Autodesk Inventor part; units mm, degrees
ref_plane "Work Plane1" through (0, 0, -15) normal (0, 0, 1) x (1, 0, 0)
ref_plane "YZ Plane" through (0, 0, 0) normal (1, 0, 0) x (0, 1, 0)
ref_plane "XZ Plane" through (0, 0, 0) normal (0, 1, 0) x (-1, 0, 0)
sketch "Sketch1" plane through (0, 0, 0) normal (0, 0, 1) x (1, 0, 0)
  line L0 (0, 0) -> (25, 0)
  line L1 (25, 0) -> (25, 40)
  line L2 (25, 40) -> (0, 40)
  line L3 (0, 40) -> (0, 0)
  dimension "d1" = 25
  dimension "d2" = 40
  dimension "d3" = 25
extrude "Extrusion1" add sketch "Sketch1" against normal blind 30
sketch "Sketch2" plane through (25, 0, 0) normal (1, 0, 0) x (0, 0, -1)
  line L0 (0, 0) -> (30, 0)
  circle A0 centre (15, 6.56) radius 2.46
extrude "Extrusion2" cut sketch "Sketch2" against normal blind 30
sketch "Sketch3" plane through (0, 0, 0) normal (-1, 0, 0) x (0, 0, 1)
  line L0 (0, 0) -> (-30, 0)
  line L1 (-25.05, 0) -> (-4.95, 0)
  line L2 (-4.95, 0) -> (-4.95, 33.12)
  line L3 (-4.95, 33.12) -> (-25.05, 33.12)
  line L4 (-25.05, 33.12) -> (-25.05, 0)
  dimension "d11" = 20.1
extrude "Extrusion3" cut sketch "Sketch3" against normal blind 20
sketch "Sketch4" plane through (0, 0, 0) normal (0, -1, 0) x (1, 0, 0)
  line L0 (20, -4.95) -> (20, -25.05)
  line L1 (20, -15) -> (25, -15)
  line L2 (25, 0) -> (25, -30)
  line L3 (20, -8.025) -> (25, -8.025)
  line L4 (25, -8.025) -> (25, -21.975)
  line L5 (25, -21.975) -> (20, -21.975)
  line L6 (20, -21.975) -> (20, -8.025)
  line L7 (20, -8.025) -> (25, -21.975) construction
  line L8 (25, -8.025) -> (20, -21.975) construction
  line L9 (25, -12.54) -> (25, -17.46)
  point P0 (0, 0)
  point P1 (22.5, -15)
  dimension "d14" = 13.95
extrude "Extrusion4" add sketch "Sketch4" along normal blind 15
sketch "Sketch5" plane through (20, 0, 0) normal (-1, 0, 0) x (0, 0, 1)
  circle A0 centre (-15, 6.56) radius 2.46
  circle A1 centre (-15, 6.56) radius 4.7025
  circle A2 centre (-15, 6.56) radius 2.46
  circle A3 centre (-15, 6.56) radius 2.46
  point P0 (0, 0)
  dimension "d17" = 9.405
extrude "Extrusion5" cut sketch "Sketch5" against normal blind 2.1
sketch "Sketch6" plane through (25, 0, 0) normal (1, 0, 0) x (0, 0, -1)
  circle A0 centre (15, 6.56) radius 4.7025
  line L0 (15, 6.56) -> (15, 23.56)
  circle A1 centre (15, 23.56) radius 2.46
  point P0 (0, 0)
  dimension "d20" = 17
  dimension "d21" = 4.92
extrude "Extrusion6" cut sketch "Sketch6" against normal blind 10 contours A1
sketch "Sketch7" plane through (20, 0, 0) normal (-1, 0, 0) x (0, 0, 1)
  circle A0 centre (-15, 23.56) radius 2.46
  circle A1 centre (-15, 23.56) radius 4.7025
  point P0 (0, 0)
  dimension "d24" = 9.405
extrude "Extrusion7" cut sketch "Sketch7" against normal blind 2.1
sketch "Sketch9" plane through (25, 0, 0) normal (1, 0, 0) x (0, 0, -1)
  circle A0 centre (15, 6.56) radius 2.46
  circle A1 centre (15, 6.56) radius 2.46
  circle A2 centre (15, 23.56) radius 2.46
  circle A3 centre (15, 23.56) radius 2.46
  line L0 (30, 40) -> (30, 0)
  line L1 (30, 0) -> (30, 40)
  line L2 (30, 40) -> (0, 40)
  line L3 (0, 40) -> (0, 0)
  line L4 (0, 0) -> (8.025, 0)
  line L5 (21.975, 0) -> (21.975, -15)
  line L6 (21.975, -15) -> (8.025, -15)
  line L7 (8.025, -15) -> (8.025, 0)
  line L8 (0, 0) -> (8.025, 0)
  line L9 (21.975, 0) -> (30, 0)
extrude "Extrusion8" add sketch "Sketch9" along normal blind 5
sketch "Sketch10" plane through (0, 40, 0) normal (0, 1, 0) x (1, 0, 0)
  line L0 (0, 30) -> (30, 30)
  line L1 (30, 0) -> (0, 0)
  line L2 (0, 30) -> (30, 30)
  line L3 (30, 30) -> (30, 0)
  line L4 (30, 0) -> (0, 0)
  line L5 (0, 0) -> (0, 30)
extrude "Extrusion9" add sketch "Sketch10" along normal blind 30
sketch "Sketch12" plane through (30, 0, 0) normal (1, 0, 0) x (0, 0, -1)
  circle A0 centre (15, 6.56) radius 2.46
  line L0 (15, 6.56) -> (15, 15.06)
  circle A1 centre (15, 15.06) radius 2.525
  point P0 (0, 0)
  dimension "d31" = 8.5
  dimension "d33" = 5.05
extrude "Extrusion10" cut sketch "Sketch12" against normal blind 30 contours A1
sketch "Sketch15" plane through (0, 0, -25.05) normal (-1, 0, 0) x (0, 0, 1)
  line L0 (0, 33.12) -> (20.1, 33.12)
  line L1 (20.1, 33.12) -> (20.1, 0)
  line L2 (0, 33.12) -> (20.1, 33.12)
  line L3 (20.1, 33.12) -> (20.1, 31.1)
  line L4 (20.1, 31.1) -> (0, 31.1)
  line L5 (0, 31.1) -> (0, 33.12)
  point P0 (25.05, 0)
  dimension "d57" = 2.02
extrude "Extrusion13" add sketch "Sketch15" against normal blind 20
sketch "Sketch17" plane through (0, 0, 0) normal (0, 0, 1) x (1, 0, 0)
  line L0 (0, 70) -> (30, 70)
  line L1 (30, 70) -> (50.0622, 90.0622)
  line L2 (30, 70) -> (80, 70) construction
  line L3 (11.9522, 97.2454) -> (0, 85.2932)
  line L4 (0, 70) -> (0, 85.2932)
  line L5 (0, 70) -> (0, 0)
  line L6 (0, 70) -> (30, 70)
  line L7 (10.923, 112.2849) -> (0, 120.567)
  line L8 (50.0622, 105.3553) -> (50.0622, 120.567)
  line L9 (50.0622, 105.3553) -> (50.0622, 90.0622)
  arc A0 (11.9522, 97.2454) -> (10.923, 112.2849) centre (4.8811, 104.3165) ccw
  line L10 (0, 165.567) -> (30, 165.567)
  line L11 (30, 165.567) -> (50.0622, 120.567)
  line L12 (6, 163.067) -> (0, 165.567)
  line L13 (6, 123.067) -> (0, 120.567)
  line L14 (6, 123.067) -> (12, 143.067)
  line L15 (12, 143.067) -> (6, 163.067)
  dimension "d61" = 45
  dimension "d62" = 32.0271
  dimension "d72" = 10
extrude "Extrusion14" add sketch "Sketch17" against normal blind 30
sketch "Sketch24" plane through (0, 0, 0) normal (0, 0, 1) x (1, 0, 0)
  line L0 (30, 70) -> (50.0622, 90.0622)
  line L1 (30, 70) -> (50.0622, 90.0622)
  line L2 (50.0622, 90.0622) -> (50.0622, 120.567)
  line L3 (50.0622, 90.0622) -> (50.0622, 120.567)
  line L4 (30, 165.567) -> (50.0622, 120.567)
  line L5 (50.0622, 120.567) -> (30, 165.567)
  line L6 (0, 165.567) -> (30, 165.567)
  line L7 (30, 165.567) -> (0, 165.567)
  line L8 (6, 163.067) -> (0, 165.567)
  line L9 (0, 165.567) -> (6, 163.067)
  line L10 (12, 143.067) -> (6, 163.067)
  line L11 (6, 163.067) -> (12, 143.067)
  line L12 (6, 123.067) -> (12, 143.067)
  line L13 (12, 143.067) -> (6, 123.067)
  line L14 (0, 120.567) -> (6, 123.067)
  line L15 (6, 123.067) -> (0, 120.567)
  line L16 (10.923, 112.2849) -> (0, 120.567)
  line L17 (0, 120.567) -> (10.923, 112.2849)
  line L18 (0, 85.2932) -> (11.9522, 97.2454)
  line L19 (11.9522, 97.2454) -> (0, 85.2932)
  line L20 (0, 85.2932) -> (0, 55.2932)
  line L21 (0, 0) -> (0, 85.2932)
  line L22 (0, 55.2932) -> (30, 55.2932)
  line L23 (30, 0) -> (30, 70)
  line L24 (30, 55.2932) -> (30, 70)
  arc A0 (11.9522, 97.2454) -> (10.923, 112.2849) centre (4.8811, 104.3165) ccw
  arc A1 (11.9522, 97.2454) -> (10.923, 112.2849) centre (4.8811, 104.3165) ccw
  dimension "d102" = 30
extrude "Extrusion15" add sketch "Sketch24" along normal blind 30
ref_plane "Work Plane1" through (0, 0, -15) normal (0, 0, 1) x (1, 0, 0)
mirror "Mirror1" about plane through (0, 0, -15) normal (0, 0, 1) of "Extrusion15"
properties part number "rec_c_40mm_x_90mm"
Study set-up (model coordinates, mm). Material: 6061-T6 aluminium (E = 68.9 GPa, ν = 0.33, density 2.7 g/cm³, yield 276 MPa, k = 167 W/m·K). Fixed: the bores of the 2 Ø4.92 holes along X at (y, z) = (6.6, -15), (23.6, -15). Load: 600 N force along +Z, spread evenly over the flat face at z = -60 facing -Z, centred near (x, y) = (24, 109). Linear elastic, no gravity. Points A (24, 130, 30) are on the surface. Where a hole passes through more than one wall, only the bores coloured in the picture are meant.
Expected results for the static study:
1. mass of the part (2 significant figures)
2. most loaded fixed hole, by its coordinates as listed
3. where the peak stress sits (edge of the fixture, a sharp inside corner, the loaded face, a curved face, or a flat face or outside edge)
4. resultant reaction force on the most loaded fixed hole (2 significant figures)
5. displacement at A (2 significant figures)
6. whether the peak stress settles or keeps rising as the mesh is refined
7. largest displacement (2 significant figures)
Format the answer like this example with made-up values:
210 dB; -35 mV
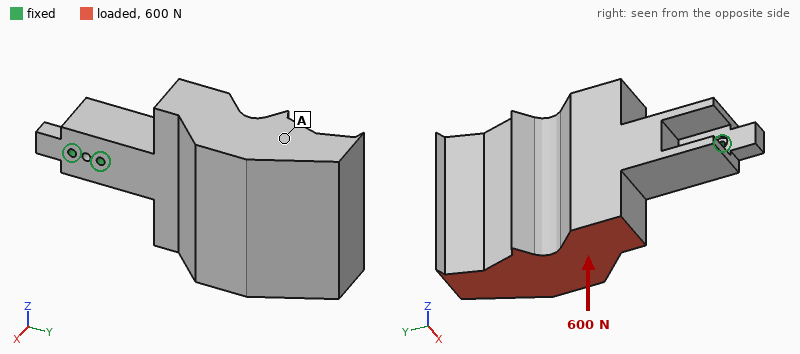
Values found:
1.0 kg; (23.6, -15); edge of the fixture; 2.8 kN; 0.12 mm; keeps rising; 0.16 mm
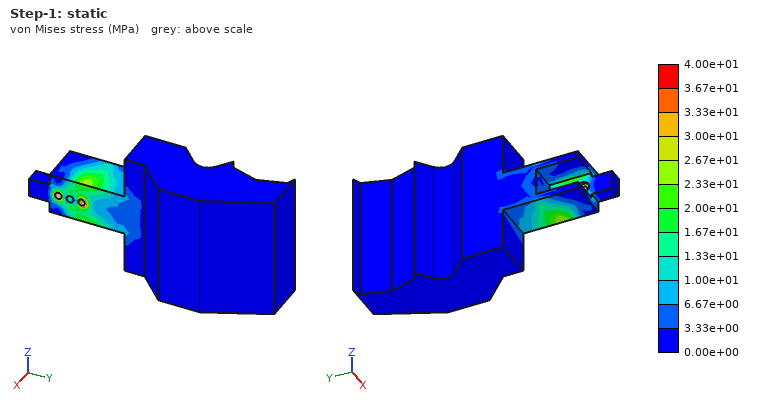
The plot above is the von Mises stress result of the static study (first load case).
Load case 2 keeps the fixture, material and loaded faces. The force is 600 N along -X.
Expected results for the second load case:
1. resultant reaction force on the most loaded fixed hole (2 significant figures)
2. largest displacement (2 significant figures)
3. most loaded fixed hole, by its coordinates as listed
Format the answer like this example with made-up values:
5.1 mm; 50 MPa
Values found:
2.6 kN; 0.27 mm; (23.6, -15)
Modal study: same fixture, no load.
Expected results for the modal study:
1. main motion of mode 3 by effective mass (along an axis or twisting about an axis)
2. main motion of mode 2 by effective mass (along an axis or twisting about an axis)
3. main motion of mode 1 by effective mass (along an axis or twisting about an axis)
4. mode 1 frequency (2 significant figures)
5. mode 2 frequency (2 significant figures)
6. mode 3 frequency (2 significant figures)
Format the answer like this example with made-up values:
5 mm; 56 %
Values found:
twisting about Y; along Z; along X; 350 Hz; 380 Hz; 760 Hz
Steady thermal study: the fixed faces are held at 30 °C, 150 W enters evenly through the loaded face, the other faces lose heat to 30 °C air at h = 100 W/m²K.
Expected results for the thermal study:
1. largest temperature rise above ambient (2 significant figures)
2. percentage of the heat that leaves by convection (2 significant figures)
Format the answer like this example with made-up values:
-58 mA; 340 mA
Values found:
38 K; 66 %
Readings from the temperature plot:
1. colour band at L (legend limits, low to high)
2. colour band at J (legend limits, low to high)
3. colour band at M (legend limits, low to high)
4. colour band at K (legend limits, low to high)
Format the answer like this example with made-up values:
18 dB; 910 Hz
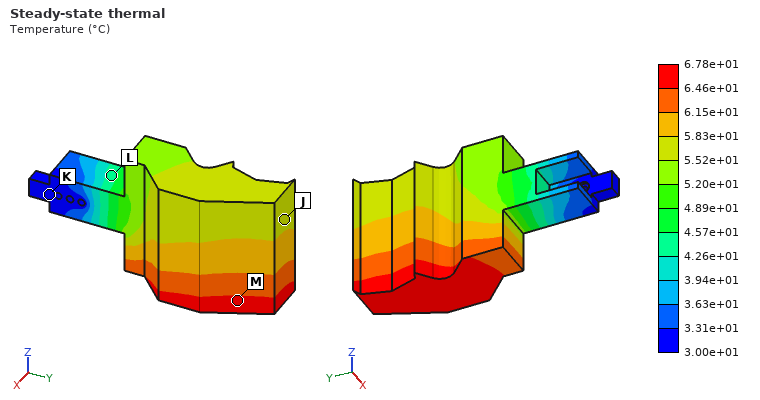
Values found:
4.26e+01 to 4.57e+01 °C; 5.52e+01 to 5.83e+01 °C; 6.46e+01 to 6.78e+01 °C; 3.00e+01 to 3.31e+01 °C
